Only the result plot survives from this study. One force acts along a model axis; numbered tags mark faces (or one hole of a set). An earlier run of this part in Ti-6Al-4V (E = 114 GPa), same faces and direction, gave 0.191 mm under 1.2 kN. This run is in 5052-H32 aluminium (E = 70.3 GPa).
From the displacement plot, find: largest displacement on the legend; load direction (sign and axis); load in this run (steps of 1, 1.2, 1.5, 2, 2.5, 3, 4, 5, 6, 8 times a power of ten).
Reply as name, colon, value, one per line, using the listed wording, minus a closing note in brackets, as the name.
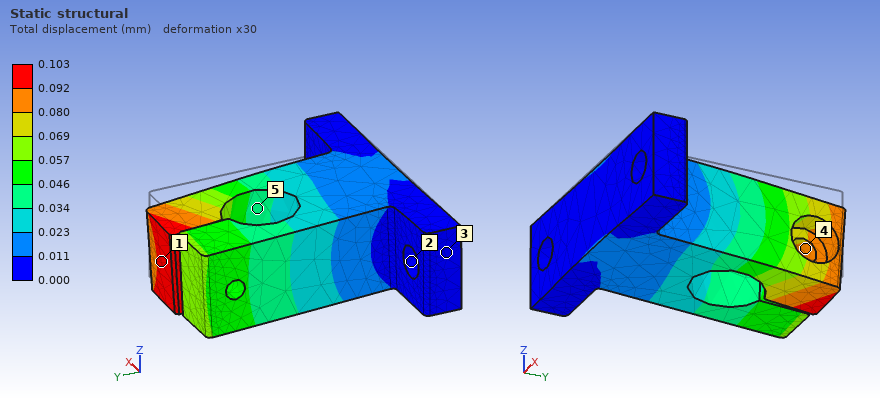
largest displacement on the legend: 0.103 mm
load direction: -Z
load in this run: 400 N
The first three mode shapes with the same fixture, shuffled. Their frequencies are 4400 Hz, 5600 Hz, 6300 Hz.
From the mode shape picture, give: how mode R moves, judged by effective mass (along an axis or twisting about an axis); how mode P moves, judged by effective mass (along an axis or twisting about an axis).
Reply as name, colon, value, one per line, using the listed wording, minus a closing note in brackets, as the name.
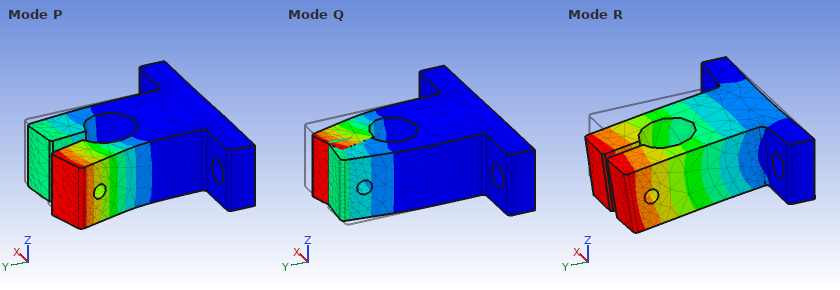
how mode R moves, judged by effective mass: along Z
how mode P moves, judged by effective mass: along X
